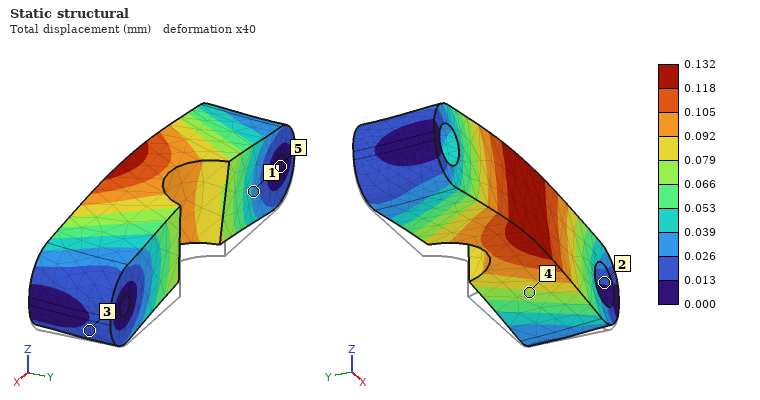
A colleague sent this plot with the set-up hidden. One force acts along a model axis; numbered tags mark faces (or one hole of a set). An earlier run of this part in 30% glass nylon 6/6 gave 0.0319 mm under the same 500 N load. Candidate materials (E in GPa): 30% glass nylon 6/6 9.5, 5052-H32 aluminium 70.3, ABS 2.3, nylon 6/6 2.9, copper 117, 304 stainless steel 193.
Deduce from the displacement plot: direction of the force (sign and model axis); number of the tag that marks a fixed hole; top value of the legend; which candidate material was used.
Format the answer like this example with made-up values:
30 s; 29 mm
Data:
+Z; 5; 0.132 mm; ABS
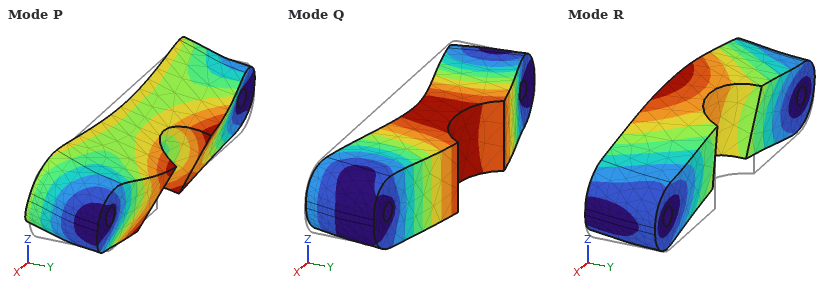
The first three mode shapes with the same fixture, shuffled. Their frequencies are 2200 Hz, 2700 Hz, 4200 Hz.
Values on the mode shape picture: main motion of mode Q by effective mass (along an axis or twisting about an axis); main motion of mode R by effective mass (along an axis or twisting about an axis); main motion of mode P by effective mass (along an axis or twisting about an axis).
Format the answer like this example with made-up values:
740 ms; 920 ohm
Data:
along Y; along Z; twisting about X
